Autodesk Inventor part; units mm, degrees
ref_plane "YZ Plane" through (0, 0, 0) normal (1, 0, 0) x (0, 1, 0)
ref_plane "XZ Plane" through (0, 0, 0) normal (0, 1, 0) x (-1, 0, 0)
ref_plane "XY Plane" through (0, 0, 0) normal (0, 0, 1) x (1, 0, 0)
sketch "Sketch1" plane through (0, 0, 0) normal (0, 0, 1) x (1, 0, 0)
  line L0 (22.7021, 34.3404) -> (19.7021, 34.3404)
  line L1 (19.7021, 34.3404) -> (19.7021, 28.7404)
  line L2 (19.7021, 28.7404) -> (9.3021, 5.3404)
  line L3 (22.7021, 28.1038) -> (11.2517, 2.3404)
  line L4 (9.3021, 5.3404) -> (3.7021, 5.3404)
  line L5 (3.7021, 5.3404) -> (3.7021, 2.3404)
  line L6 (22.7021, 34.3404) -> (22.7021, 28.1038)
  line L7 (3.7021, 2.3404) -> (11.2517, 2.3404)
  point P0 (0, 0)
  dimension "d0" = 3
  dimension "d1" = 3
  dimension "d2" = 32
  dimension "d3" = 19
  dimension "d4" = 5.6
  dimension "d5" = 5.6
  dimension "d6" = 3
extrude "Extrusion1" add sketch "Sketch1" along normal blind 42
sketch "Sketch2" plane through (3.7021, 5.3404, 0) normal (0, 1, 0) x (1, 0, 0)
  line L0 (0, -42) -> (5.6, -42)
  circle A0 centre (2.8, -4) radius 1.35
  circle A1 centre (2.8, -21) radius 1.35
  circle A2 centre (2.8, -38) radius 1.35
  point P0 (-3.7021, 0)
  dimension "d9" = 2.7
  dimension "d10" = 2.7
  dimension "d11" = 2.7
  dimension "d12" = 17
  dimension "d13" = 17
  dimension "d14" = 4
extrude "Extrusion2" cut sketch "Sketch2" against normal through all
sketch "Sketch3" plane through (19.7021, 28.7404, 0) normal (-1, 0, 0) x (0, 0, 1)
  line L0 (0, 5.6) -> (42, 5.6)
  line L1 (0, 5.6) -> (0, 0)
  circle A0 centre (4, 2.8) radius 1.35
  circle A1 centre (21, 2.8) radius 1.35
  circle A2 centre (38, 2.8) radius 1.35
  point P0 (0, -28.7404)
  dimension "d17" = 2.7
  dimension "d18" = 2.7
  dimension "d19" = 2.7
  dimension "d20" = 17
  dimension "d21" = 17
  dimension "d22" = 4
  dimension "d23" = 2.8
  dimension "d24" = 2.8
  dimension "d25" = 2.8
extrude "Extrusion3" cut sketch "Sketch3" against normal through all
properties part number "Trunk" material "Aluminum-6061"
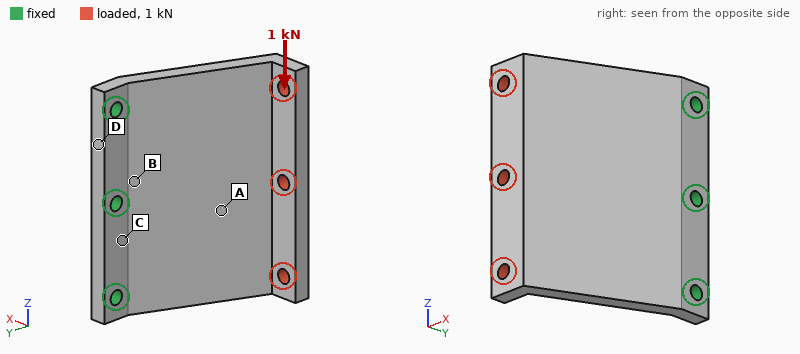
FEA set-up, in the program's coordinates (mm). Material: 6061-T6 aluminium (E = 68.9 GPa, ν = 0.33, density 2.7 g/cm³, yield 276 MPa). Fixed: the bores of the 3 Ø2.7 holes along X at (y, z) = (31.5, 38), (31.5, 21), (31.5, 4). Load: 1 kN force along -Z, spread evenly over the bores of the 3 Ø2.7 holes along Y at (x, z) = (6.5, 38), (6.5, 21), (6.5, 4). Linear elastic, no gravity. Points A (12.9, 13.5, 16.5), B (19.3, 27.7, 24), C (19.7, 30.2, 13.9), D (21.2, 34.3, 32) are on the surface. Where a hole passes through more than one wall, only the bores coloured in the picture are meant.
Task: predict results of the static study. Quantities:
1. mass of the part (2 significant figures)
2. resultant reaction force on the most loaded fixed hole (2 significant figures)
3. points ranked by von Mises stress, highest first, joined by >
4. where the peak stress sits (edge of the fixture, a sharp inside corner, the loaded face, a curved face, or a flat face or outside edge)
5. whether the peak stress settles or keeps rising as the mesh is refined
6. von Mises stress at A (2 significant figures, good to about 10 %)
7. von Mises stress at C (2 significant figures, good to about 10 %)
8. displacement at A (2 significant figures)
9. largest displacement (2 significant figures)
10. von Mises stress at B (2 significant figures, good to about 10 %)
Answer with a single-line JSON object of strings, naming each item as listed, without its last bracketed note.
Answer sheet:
{"mass of the part": "13 g", "resultant reaction force on the most loaded fixed hole": "940 N", "points ranked by von Mises stress, highest first, joined by >": "A > B > C > D", "where the peak stress sits": "edge of the fixture", "whether the peak stress settles or keeps rising as the mesh is refined": "keeps rising", "von Mises stress at A": "56 MPa", "von Mises stress at C": "23 MPa", "displacement at A": "0.028 mm", "largest displacement": "0.17 mm", "von Mises stress at B": "37 MPa"}
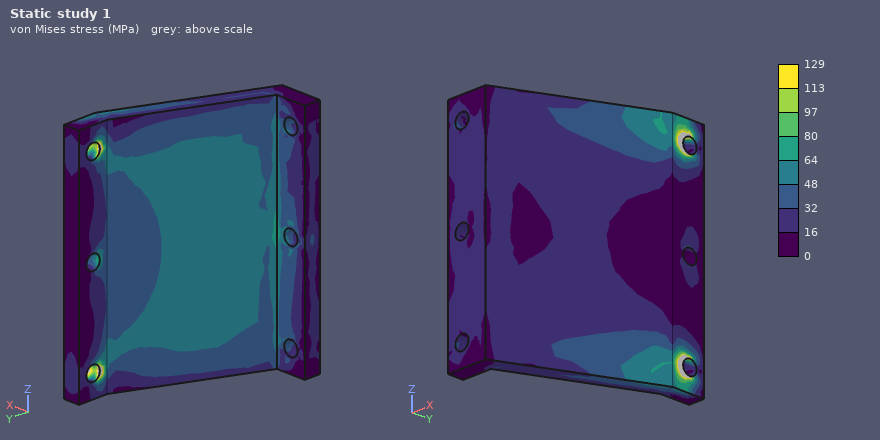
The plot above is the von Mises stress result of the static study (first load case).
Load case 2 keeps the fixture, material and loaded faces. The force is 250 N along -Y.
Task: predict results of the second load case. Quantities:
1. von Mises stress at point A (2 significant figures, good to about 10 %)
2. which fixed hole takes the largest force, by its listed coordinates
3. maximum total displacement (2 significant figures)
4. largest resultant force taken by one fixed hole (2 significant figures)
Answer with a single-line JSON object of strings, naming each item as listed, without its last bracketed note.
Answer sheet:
{"von Mises stress at point A": "29 MPa", "which fixed hole takes the largest force, by its listed coordinates": "(31.5, 21)", "maximum total displacement": "0.26 mm", "largest resultant force taken by one fixed hole": "140 N"}
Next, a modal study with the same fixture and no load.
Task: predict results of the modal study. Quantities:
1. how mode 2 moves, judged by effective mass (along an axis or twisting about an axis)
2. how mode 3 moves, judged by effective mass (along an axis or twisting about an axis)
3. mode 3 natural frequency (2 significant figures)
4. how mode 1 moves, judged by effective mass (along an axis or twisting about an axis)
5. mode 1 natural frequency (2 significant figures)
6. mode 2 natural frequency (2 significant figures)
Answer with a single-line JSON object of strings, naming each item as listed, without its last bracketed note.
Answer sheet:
{"how mode 2 moves, judged by effective mass": "twisting about Y", "how mode 3 moves, judged by effective mass": "along X", "mode 3 natural frequency": "11 kHz", "how mode 1 moves, judged by effective mass": "along X", "mode 1 natural frequency": "1900 Hz", "mode 2 natural frequency": "4100 Hz"}
